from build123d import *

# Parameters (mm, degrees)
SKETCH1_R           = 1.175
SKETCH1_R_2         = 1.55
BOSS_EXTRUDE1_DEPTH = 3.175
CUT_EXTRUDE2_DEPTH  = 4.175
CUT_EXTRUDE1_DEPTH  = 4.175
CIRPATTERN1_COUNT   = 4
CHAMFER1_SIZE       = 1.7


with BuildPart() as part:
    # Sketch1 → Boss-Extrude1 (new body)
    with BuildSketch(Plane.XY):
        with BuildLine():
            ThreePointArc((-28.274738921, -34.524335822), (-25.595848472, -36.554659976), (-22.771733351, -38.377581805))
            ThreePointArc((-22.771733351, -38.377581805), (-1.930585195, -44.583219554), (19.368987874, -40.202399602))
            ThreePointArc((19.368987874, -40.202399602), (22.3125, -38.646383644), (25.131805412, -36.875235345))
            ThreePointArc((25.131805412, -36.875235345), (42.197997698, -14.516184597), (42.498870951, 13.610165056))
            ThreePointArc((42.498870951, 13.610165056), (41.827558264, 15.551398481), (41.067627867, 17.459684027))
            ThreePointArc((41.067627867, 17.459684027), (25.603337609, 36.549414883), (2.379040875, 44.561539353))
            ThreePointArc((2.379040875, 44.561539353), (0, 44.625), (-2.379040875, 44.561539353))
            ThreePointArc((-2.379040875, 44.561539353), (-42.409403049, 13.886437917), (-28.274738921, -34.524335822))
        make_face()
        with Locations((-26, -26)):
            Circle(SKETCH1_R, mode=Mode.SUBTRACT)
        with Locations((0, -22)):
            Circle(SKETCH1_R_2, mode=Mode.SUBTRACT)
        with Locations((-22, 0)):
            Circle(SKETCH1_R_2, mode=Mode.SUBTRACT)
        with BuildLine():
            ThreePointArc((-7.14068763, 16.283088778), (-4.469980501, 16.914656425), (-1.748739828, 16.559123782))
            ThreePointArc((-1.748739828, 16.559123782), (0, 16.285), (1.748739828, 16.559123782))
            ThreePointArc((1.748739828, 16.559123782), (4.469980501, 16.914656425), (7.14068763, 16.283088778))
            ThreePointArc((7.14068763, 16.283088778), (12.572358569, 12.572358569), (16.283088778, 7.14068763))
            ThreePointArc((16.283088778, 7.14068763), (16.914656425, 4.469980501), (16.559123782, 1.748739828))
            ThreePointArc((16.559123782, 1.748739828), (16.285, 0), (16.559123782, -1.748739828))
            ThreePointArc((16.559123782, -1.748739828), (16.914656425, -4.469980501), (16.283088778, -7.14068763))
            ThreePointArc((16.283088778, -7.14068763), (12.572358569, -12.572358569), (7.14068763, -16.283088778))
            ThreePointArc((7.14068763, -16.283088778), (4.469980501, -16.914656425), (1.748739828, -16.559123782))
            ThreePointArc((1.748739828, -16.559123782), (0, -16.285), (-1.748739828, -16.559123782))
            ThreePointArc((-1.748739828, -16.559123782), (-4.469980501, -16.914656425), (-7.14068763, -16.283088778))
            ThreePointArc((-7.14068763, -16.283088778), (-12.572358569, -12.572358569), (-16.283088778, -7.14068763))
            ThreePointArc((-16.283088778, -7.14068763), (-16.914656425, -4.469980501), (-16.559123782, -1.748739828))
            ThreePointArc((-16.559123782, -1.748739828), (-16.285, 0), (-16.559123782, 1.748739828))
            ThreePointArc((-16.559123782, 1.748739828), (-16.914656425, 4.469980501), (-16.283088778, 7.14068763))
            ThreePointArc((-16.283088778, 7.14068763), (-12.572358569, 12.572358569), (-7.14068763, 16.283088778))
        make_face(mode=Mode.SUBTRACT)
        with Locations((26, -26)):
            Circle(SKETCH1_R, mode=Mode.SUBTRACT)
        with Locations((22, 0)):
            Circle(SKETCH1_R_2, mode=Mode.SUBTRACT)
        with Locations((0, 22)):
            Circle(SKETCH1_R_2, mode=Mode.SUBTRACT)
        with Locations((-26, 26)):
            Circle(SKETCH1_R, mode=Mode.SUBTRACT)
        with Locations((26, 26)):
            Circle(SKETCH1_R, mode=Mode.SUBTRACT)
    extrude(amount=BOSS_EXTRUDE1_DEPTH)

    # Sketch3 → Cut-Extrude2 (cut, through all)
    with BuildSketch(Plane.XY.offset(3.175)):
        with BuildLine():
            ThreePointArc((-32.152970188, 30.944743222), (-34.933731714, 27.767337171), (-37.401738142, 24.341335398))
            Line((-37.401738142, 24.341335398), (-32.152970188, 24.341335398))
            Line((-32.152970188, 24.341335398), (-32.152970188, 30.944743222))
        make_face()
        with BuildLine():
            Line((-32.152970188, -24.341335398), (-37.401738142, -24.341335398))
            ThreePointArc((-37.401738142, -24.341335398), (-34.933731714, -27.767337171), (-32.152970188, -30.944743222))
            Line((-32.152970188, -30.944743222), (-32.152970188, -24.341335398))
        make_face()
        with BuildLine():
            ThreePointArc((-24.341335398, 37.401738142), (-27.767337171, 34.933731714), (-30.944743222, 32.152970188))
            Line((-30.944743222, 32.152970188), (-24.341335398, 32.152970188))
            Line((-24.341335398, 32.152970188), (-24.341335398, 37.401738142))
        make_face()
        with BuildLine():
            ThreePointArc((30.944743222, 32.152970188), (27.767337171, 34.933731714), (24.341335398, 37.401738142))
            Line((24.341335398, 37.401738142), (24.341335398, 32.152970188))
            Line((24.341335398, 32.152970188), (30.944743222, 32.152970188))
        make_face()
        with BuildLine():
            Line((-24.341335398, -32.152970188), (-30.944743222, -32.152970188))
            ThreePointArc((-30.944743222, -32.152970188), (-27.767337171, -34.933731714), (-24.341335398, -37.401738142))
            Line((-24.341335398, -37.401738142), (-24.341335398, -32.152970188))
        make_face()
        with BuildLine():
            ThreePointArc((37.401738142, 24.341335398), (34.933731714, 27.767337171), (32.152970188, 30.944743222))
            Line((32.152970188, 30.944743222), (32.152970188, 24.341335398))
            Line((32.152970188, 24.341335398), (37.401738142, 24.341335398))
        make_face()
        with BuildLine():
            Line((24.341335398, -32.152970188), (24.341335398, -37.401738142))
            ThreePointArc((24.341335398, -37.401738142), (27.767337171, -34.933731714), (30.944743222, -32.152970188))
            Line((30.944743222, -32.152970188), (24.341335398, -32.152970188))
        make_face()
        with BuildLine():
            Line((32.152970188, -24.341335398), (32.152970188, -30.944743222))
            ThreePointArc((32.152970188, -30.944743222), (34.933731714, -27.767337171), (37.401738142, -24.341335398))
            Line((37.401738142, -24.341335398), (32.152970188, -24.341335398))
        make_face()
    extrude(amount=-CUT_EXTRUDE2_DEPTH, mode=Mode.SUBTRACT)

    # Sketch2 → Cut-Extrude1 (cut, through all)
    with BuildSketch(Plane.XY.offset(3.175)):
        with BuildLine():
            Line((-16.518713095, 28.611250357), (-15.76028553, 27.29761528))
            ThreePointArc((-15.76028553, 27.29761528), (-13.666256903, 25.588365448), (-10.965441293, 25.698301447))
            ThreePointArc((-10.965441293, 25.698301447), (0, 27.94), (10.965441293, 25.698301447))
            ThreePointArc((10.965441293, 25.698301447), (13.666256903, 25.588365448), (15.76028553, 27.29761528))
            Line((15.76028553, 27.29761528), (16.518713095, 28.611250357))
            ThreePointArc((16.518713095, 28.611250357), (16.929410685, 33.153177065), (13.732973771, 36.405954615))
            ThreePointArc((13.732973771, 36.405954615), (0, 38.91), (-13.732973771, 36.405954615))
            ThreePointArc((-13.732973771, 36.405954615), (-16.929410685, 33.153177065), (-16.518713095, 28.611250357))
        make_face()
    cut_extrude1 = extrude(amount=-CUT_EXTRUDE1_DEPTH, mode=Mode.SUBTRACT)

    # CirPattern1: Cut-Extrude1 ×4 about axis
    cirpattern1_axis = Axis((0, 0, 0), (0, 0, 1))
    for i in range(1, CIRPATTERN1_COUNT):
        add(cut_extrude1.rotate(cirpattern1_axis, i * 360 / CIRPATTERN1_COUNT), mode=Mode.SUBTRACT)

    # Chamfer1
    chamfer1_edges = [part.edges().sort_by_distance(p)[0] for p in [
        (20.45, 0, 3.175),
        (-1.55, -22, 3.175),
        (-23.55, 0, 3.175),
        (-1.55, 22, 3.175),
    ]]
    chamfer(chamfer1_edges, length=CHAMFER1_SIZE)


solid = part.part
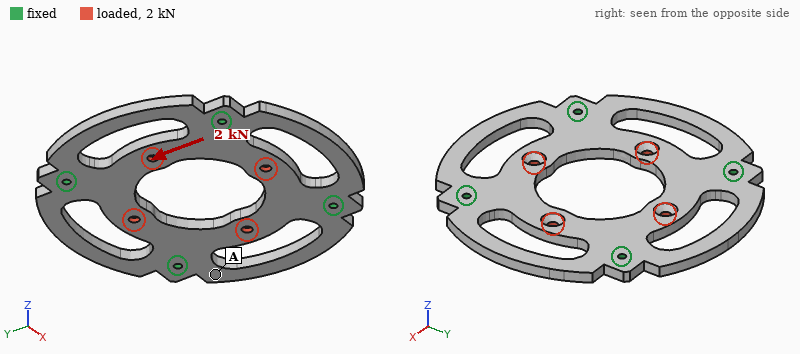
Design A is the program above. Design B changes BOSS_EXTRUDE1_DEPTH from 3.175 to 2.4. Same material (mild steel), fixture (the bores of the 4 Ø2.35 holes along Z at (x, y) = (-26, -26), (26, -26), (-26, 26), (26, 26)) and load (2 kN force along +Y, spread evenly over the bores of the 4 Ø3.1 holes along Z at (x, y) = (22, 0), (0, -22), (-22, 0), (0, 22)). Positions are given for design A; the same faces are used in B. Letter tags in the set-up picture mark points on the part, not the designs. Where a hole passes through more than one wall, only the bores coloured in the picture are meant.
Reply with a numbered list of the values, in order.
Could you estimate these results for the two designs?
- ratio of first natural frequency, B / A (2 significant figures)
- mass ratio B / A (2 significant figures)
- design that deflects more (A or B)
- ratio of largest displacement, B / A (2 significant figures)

1. 0.78
2. 0.75
3. B
4. 1.6
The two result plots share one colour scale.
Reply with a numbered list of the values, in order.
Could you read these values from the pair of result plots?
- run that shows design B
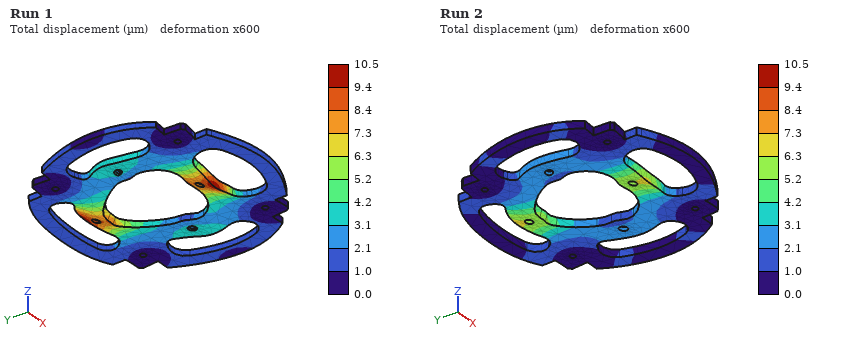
1. Run 1
